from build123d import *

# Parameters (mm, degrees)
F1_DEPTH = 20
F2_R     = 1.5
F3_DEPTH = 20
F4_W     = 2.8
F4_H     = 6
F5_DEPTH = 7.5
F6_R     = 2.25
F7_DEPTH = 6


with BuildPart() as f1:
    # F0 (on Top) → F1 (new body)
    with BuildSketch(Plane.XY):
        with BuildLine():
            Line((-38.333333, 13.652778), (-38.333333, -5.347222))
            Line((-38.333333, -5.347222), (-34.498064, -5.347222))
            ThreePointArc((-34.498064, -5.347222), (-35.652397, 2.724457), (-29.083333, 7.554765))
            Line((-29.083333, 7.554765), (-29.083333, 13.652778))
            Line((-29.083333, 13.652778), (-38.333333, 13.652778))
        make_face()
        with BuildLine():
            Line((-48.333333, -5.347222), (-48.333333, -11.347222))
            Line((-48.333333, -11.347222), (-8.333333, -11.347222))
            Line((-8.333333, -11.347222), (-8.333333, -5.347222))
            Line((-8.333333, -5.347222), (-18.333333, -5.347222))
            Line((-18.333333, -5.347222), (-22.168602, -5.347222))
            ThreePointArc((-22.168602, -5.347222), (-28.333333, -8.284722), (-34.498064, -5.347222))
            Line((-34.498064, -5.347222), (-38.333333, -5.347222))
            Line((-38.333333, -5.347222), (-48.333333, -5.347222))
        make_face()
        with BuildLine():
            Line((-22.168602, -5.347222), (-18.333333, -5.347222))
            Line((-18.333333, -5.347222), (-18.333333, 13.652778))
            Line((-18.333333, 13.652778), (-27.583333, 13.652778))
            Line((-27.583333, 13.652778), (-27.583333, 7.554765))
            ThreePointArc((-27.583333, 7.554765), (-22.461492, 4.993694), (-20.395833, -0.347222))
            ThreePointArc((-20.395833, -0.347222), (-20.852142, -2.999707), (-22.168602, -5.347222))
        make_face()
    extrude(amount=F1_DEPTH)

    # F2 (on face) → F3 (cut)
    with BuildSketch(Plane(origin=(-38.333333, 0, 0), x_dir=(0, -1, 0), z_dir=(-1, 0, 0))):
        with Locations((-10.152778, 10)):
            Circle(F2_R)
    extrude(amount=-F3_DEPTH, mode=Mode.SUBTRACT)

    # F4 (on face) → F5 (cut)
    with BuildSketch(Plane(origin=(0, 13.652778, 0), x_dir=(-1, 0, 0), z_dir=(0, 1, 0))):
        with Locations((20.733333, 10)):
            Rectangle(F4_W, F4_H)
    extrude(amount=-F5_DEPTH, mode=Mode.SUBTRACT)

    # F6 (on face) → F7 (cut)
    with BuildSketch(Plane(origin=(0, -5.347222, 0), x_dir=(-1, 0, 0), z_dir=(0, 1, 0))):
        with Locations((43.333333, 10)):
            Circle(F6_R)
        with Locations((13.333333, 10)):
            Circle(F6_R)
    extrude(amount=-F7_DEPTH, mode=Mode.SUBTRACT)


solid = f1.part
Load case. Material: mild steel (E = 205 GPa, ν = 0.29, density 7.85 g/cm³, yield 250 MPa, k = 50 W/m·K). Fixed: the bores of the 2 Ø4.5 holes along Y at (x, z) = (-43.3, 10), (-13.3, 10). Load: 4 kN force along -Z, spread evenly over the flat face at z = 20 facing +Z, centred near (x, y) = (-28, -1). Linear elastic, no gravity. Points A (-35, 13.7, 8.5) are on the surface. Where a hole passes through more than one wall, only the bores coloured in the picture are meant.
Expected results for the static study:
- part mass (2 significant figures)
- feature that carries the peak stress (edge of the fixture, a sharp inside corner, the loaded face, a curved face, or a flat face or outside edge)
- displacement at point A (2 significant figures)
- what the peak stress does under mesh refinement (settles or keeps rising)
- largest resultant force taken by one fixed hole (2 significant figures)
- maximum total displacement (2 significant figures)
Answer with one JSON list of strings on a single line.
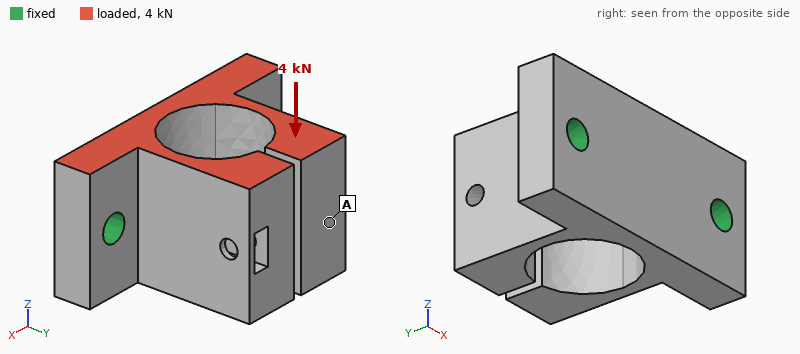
["61 g", "edge of the fixture", "29 µm", "keeps rising", "2.0 kN", "38 µm"]
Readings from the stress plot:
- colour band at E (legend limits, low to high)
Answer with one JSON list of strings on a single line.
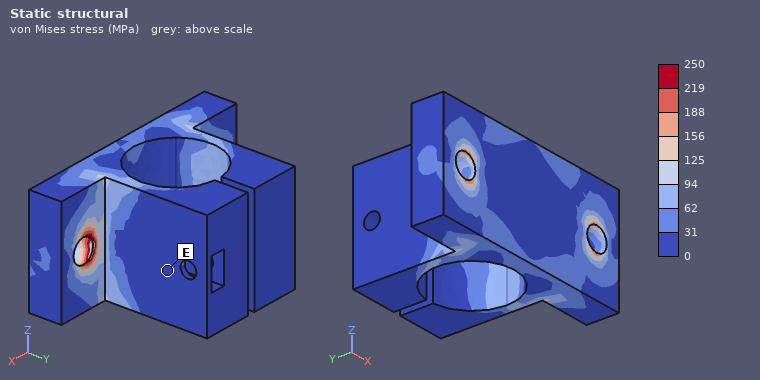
["0 to 31 MPa"]
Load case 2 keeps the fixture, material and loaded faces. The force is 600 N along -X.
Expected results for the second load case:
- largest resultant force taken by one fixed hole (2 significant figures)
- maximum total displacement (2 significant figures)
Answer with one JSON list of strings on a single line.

["360 N", "48 µm"]
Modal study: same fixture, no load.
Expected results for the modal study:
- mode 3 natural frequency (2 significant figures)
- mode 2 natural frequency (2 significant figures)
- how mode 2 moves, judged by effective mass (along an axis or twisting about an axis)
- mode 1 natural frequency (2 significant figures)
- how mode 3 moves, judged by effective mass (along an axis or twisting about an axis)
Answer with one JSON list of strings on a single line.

["7600 Hz", "2900 Hz", "along X", "2800 Hz", "along Z"]
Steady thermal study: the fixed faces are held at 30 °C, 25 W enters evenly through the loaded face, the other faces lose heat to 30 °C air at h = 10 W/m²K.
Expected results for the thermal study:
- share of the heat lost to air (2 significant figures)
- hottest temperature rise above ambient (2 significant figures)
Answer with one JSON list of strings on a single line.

["3.9 %", "48 K"]
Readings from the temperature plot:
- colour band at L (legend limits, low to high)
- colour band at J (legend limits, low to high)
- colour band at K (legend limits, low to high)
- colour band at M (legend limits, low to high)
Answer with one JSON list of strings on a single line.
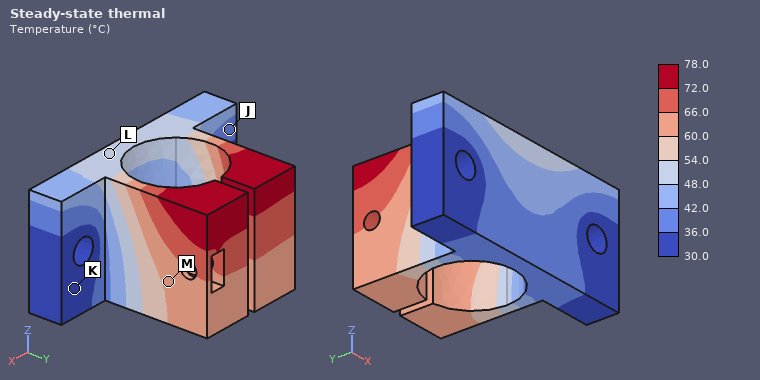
["48.0 to 54.0 °C", "36.0 to 42.0 °C", "30.0 to 36.0 °C", "60.0 to 66.0 °C"]
